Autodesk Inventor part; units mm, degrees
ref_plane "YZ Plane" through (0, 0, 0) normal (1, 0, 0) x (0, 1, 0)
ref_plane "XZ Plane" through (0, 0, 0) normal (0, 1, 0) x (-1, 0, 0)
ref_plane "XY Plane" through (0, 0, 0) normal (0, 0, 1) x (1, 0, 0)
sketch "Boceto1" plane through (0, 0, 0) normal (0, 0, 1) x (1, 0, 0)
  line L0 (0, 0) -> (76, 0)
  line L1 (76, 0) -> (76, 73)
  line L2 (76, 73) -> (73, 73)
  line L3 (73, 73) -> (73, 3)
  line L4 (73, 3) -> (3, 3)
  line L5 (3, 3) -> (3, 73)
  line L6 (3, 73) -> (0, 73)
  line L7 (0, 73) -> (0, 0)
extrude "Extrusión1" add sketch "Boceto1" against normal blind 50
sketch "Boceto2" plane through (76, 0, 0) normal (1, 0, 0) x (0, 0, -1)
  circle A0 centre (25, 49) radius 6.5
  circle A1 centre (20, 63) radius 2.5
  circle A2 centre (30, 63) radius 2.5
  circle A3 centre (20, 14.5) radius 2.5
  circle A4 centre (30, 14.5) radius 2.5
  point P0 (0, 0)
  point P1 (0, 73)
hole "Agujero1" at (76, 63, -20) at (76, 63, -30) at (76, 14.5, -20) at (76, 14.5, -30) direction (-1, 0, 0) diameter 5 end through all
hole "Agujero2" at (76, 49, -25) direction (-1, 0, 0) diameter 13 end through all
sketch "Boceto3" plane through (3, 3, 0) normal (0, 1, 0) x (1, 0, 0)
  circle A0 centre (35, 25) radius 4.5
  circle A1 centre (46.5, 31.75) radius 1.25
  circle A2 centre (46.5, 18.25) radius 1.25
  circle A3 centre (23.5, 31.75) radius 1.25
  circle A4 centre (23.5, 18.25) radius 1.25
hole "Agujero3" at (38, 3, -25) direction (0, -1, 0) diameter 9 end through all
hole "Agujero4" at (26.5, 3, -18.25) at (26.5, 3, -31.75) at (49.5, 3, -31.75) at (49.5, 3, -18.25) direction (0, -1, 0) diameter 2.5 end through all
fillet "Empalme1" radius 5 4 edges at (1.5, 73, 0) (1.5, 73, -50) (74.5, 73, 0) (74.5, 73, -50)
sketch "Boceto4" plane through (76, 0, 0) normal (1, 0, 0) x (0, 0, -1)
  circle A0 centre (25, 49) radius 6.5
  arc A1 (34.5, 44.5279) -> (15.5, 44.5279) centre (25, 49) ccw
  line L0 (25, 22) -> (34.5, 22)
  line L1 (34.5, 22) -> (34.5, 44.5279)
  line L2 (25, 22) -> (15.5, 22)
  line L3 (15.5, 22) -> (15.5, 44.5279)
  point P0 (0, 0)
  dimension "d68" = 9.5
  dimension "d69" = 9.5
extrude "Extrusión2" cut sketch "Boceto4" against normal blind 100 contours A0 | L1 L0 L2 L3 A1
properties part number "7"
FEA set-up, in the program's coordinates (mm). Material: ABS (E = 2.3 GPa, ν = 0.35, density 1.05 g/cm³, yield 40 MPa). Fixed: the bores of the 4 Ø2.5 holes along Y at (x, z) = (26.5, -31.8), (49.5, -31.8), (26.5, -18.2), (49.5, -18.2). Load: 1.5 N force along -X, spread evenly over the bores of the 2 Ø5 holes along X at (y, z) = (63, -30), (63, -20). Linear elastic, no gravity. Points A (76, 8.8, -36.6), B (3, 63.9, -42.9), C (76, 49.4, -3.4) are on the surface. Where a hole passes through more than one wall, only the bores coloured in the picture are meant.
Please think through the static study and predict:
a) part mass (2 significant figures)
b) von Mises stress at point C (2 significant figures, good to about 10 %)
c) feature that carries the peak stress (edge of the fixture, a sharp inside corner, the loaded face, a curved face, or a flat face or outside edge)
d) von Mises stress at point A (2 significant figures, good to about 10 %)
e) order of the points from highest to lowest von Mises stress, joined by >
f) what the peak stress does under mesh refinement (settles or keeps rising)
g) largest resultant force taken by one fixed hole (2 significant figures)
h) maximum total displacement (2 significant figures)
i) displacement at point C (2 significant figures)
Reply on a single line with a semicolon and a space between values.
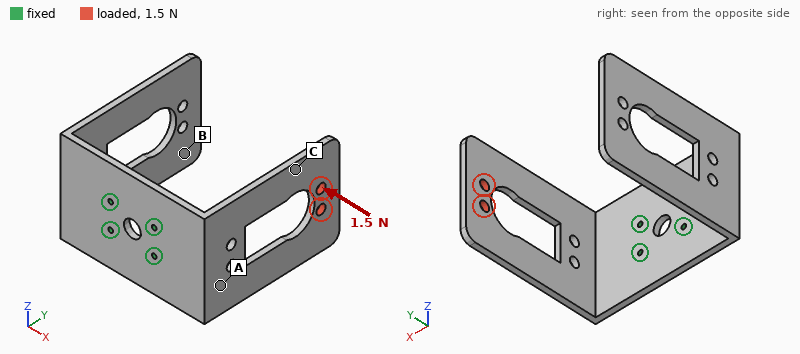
29 g; 0.46 MPa; edge of the fixture; 0.99 MPa; A > C > B; keeps rising; 1.1 N; 1.3 mm; 0.77 mm
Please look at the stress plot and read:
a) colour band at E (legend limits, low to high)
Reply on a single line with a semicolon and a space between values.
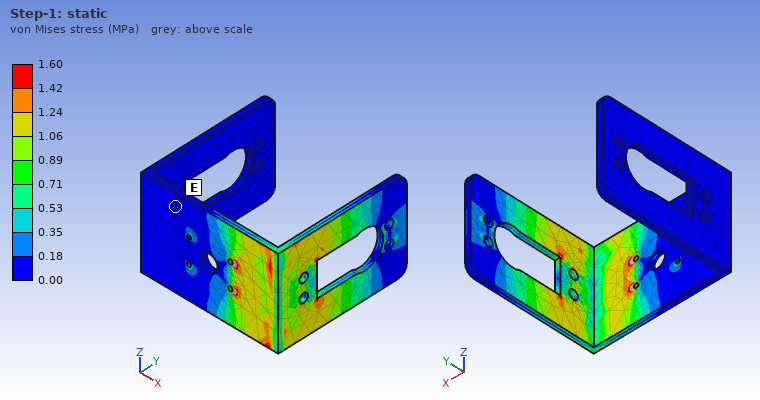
0.00 to 0.18 MPa
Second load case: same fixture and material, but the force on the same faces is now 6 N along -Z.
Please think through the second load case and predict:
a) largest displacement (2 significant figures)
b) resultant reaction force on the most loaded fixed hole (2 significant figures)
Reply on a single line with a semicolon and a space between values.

1.1 mm; 21 N
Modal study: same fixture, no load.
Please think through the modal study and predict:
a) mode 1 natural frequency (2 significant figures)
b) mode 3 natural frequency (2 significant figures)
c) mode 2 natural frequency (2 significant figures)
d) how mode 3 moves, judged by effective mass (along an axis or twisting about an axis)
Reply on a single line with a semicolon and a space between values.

96 Hz; 180 Hz; 98 Hz; twisting about Y
